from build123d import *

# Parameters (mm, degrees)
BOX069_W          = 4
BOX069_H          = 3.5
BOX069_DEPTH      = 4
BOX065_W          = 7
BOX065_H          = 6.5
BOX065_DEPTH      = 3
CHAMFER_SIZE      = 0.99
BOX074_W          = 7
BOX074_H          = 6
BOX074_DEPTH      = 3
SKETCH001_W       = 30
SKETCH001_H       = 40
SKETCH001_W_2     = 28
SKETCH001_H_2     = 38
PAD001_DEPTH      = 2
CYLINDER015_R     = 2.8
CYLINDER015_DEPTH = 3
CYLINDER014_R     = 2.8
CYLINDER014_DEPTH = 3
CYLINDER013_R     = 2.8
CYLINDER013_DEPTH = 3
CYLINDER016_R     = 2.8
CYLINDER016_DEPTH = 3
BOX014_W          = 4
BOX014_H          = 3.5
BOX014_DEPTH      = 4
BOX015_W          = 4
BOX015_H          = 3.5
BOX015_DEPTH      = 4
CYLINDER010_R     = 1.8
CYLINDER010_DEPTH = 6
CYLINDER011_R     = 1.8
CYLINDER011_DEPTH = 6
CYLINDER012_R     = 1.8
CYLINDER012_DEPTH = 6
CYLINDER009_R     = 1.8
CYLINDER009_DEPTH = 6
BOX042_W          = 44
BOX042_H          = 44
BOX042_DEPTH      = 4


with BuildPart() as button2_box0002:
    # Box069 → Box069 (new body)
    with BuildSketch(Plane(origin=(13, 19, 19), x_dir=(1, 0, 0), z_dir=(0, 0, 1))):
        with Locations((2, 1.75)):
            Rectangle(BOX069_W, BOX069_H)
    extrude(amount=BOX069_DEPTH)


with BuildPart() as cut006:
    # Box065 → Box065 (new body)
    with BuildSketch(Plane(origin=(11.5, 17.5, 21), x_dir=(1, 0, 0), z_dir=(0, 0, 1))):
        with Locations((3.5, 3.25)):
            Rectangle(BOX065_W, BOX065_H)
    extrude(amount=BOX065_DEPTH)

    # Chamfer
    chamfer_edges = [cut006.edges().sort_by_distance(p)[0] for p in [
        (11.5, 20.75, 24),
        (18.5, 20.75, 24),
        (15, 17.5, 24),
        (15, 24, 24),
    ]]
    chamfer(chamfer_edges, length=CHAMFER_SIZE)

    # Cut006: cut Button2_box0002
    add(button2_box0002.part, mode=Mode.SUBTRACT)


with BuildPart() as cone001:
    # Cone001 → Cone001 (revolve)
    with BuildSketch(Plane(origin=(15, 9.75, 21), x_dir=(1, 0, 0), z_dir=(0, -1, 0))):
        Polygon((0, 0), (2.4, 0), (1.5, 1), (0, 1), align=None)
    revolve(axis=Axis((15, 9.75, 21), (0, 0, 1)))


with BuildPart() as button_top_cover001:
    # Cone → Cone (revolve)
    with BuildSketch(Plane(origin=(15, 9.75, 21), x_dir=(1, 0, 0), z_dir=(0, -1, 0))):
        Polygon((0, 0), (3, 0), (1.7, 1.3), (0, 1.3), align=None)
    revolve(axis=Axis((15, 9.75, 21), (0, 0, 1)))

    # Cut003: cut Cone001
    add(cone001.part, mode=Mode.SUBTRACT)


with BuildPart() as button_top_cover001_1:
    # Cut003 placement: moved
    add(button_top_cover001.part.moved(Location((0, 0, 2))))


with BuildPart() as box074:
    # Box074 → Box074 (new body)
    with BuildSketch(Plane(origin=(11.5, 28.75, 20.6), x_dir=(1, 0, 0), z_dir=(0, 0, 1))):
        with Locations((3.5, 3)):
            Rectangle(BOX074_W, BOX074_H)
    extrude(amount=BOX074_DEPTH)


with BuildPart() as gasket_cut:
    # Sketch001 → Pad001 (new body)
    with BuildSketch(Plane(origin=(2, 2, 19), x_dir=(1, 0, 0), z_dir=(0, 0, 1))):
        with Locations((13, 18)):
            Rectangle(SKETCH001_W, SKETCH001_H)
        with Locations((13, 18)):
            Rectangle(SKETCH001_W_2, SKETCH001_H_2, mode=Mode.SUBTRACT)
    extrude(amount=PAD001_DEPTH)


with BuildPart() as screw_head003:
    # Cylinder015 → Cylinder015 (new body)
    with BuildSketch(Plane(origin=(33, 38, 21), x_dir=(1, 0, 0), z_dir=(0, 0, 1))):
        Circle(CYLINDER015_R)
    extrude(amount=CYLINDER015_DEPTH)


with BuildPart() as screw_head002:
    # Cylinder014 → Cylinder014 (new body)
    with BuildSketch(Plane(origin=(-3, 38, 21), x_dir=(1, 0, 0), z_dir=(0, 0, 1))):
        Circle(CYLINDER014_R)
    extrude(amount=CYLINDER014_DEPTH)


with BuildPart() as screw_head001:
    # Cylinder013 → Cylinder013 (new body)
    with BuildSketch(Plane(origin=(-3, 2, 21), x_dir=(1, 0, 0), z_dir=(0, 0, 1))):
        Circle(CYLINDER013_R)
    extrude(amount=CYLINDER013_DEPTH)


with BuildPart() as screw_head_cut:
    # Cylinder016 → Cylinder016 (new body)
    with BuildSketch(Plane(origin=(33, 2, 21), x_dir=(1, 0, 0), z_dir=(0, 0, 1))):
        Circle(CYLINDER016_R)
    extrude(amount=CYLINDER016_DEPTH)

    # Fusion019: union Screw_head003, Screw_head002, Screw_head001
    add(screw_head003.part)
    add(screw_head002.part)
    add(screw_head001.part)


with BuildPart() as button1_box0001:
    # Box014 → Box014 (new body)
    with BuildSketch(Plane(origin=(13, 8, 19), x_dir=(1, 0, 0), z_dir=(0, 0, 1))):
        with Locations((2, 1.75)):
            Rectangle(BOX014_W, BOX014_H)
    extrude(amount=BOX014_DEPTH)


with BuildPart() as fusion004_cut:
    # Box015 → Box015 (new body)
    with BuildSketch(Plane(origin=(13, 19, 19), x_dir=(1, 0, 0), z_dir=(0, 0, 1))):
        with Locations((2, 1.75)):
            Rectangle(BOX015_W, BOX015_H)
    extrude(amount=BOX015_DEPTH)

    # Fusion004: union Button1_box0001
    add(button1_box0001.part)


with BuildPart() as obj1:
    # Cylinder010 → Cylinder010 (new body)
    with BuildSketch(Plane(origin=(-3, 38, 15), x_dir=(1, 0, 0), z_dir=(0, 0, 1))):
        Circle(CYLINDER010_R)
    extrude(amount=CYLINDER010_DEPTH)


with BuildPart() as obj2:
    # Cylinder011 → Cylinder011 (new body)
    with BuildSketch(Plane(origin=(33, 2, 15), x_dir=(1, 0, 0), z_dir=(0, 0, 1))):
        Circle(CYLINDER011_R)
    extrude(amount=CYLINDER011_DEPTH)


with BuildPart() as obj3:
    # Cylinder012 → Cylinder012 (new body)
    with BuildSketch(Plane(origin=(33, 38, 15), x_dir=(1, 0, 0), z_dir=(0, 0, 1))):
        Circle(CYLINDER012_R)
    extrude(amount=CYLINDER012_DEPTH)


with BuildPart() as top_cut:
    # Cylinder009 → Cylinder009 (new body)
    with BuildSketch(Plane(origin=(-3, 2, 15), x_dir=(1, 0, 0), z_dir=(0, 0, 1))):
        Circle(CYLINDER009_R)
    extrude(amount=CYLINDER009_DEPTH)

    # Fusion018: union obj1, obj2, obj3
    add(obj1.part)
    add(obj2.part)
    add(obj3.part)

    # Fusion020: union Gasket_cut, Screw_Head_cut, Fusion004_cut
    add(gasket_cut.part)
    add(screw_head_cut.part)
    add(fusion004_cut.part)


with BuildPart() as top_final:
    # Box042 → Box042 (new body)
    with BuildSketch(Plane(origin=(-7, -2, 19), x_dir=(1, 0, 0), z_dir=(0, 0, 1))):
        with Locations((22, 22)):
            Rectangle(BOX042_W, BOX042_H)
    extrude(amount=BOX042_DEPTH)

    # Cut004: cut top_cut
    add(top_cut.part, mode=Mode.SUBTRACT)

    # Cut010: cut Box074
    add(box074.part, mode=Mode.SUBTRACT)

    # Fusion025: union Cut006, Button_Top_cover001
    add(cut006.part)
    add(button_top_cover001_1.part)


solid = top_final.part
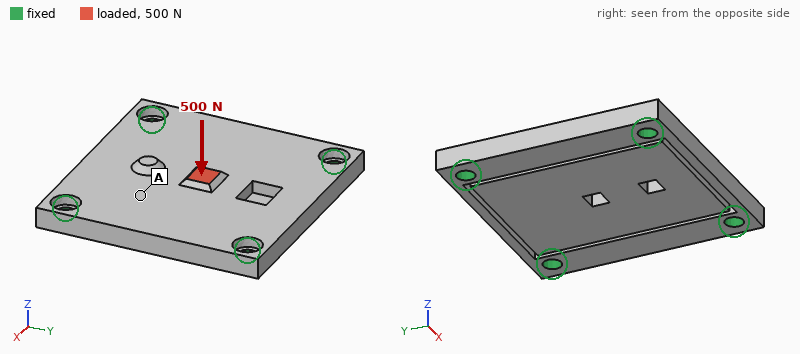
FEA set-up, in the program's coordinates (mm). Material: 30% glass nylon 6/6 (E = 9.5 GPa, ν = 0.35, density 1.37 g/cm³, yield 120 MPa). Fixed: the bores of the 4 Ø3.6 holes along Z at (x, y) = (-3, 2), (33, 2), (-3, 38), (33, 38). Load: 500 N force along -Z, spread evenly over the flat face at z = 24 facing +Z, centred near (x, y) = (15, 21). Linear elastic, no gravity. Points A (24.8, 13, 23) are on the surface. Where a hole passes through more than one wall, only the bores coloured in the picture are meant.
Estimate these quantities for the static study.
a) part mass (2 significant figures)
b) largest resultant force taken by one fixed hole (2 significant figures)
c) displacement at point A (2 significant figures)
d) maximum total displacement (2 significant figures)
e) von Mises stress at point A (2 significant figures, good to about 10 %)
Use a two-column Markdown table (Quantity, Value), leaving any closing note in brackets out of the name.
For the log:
| Quantity | Value |
|---|---|
| part mass | 9.6 g |
| largest resultant force taken by one fixed hole | 170 N |
| displacement at point A | 0.14 mm |
| maximum total displacement | 0.25 mm |
| von Mises stress at point A | 14 MPa |
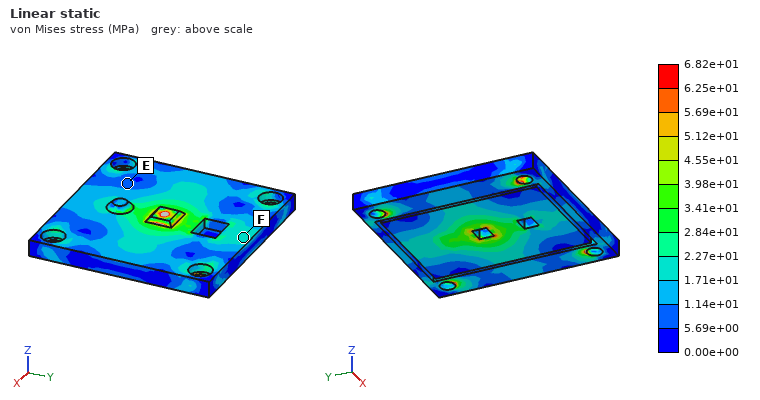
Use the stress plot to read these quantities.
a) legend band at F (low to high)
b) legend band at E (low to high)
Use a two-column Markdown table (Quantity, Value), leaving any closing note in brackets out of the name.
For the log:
| Quantity | Value |
|---|---|
| legend band at F | 1.71e+01 to 2.27e+01 MPa |
| legend band at E | 5.69e+00 to 1.14e+01 MPa |
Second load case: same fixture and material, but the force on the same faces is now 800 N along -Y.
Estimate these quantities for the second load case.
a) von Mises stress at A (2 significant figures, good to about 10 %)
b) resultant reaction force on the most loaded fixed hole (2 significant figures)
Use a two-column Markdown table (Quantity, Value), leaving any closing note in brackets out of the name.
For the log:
| Quantity | Value |
|---|---|
| von Mises stress at A | 10 MPa |
| resultant reaction force on the most loaded fixed hole | 220 N |
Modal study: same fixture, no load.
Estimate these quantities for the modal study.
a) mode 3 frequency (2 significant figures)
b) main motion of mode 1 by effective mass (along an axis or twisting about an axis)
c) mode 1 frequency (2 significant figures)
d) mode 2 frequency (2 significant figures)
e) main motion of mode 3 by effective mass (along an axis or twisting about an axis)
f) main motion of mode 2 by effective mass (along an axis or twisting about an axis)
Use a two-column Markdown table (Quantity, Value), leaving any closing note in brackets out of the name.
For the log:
| Quantity | Value |
|---|---|
| mode 3 frequency | 7400 Hz |
| main motion of mode 1 by effective mass | along Z |
| mode 1 frequency | 4400 Hz |
| mode 2 frequency | 6900 Hz |
| main motion of mode 3 by effective mass | twisting about Y |
| main motion of mode 2 by effective mass | twisting about X |
